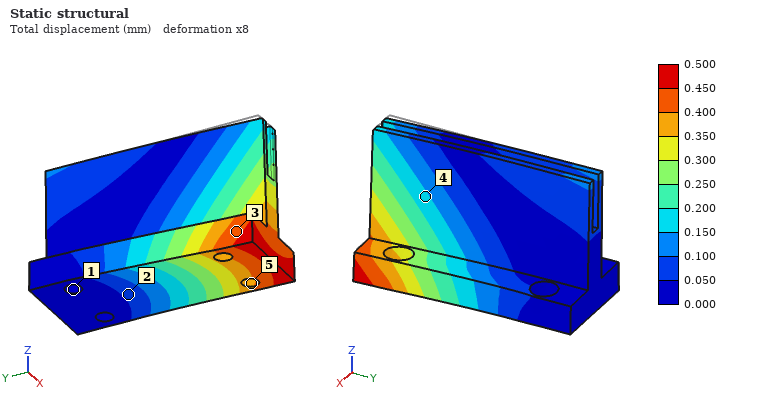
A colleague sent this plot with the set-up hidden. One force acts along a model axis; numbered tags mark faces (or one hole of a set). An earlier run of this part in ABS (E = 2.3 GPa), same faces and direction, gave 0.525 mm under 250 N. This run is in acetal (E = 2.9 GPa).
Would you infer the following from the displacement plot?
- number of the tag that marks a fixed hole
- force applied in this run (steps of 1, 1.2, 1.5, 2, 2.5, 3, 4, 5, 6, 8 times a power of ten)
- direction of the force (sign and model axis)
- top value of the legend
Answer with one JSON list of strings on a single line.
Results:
["1", "300 N", "+X", "0.500 mm"]
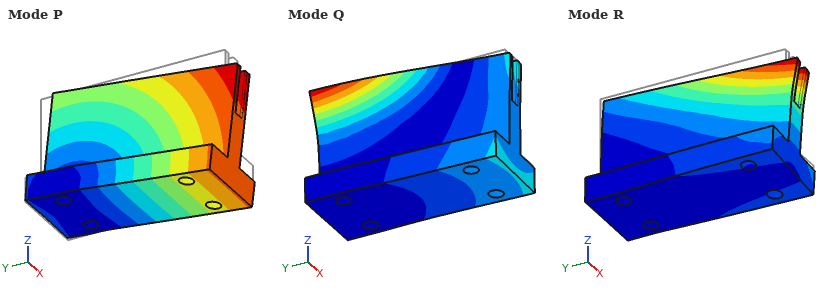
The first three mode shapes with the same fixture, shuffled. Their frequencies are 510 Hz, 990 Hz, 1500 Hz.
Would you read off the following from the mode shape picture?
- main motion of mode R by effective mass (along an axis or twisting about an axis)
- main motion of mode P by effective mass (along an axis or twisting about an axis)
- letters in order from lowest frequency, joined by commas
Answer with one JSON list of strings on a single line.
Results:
["along X", "along Z", "P, R, Q"]
